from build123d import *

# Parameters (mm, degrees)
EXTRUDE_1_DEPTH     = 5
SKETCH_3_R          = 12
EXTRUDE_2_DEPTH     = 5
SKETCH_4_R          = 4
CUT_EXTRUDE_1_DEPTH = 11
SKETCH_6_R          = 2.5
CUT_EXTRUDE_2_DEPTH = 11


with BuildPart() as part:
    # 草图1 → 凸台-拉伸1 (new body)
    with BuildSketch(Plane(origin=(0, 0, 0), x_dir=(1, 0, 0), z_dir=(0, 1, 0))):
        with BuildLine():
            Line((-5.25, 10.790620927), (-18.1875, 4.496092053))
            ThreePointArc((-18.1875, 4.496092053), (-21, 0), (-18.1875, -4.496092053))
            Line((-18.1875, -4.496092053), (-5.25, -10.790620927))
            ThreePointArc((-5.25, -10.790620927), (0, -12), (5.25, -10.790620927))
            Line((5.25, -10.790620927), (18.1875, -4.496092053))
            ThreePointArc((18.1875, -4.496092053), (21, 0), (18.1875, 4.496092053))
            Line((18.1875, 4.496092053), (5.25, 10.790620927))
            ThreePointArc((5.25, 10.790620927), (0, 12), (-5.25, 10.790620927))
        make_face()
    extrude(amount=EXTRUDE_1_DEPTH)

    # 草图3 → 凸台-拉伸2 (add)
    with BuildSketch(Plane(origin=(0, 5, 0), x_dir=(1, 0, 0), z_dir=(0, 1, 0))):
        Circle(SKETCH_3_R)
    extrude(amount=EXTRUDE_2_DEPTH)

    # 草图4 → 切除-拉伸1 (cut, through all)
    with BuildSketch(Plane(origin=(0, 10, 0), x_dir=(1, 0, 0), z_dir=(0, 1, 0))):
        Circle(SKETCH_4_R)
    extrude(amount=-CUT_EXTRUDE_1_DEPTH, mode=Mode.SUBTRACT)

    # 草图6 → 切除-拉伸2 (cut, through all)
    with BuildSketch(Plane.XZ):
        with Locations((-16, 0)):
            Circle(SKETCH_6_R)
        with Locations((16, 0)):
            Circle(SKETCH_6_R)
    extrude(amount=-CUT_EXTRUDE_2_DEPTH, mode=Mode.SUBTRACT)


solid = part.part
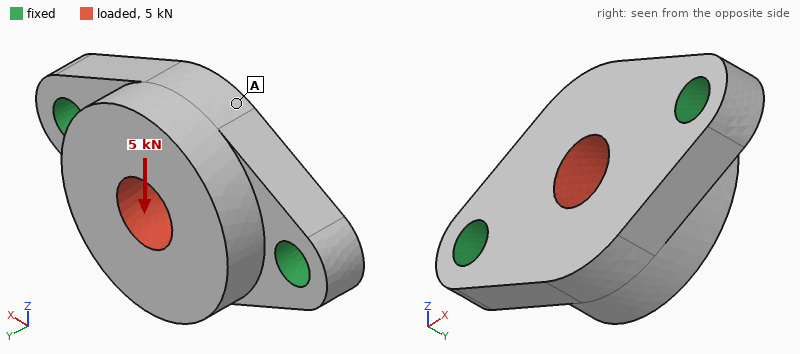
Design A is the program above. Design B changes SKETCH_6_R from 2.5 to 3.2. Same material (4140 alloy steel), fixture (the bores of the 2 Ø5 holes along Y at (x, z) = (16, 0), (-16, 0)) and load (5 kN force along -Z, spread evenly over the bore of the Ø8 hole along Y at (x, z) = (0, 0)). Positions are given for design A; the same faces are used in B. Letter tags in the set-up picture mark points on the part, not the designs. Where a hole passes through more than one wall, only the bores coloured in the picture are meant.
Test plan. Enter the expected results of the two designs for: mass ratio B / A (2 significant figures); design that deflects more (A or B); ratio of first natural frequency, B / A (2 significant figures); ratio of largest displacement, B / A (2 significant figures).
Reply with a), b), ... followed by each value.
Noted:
a) 0.97
b) A
c) 1.1
d) 0.78
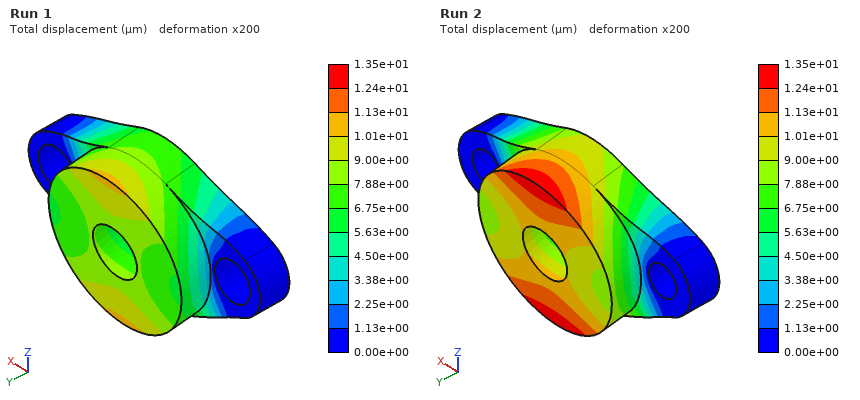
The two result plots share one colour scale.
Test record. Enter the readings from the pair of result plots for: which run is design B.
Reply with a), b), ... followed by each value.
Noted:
a) Run 1
